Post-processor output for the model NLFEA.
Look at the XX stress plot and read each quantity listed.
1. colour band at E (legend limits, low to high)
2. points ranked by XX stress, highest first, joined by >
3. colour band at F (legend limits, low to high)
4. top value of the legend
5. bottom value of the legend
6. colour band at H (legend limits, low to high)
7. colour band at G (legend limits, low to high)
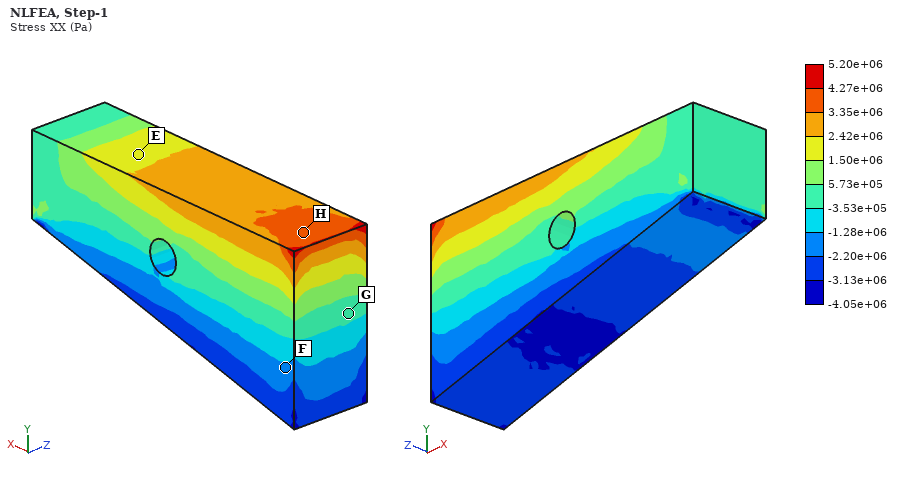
1.50e+06 to 2.42e+06 Pa
H > E > G > F
-2.20e+06 to -1.28e+06 Pa
5.20e+06 Pa
-4.05e+06 Pa
3.35e+06 to 4.27e+06 Pa
-3.53e+05 to 5.73e+05 Pa
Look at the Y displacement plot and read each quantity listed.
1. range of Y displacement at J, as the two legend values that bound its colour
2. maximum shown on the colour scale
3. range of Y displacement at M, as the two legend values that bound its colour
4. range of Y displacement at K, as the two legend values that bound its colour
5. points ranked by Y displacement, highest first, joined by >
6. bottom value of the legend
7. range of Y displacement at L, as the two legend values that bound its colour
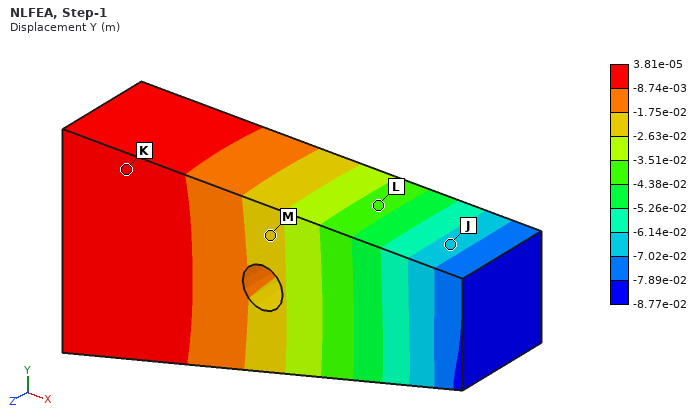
-7.02e-02 to -6.14e-02 m
3.81e-05 m
-2.63e-02 to -1.75e-02 m
-8.74e-03 to 3.81e-05 m
K > M > L > J
-8.77e-02 m
-4.38e-02 to -3.51e-02 m
